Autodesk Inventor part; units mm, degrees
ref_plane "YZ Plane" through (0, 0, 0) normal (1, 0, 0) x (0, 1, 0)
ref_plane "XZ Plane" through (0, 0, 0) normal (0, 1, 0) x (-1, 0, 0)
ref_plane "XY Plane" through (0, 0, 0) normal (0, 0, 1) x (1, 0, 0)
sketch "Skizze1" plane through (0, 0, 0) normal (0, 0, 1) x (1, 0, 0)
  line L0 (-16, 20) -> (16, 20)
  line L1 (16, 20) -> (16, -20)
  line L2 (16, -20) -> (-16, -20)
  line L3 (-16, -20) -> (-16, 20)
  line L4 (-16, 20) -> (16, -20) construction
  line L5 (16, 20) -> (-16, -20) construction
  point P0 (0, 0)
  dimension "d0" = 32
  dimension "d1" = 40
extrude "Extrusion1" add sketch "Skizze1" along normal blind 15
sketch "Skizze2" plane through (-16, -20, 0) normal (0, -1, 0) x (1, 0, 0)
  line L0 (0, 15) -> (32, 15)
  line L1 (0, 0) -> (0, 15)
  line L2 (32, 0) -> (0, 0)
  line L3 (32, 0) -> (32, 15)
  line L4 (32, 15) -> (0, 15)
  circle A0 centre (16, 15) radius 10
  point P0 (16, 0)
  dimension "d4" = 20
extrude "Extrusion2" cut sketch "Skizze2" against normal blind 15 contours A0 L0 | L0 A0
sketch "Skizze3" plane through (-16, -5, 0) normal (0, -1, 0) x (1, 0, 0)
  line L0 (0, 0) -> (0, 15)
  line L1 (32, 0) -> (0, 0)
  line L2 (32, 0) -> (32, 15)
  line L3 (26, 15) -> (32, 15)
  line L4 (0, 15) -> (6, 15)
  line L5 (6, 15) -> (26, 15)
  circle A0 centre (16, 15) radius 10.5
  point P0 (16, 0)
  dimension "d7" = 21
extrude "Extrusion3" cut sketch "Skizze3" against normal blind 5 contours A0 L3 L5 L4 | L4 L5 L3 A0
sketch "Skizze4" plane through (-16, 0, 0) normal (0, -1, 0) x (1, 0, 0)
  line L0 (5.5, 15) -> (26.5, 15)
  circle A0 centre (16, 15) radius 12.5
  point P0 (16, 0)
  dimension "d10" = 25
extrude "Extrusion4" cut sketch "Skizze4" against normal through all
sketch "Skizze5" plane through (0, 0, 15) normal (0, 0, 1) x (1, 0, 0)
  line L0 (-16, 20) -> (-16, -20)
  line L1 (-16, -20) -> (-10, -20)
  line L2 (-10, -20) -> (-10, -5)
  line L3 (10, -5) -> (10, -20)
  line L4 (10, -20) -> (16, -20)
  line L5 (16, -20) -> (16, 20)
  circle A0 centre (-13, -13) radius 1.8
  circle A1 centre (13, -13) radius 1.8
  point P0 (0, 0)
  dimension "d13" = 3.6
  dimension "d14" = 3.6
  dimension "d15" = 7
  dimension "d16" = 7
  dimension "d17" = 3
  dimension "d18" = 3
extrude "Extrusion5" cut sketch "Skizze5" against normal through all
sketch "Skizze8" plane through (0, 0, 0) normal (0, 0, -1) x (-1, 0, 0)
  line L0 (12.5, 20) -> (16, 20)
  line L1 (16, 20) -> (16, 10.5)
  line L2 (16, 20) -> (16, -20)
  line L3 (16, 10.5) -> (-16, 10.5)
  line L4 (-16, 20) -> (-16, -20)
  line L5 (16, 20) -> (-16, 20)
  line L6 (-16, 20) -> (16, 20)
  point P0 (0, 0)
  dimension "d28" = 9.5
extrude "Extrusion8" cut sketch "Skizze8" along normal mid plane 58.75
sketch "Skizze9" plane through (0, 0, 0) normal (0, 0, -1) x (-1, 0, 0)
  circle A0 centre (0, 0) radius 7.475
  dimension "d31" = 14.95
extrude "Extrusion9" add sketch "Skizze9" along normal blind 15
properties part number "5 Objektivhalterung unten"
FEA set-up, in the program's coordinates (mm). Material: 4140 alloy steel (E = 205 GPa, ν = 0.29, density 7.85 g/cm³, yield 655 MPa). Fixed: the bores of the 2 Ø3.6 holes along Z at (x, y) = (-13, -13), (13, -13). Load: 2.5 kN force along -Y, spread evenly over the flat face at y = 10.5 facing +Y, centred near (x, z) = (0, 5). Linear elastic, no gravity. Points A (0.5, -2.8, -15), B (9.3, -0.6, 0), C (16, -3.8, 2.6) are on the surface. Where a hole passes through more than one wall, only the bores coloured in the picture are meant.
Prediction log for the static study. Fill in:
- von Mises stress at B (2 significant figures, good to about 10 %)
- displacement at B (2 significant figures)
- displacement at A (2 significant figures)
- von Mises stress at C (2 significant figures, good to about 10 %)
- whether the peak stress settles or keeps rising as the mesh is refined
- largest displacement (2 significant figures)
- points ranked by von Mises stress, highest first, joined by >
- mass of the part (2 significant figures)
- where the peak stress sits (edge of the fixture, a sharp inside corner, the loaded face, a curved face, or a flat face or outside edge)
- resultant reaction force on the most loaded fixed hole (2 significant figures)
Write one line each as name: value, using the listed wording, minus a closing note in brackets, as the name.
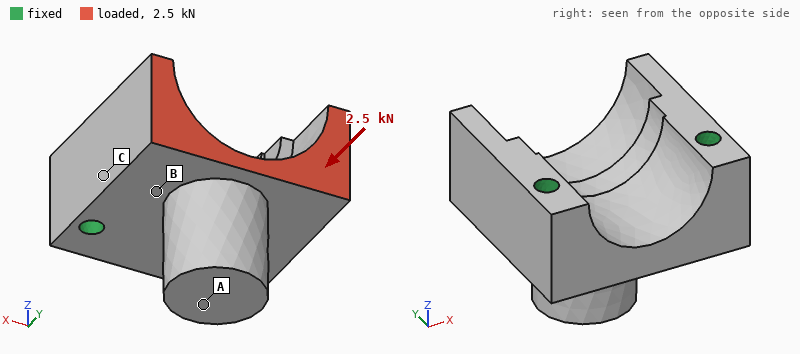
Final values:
von Mises stress at B: 8.9 MPa
displacement at B: 0.96 µm
displacement at A: 1.6 µm
von Mises stress at C: 14 MPa
whether the peak stress settles or keeps rising as the mesh is refined: keeps rising
largest displacement: 1.7 µm
points ranked by von Mises stress, highest first, joined by >: C > B > A
mass of the part: 88 g
where the peak stress sits: edge of the fixture
resultant reaction force on the most loaded fixed hole: 1.3 kN
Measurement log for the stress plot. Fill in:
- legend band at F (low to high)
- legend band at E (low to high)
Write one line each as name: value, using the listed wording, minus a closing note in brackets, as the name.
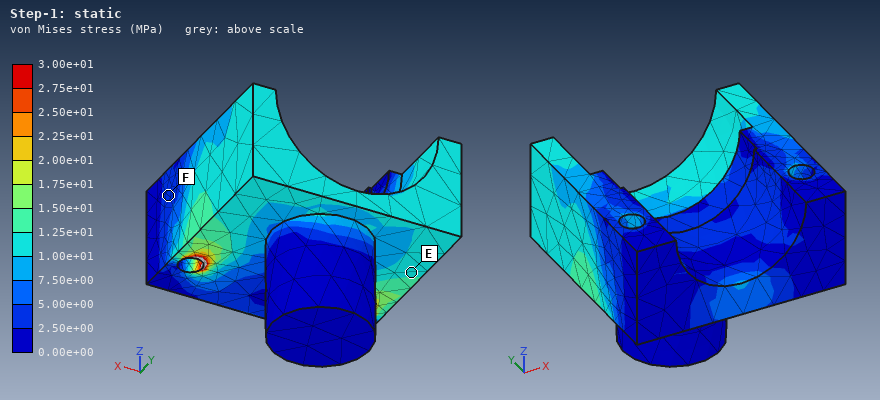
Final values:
legend band at F: 2.50e+00 to 5.00e+00 MPa
legend band at E: 1.00e+01 to 1.25e+01 MPa
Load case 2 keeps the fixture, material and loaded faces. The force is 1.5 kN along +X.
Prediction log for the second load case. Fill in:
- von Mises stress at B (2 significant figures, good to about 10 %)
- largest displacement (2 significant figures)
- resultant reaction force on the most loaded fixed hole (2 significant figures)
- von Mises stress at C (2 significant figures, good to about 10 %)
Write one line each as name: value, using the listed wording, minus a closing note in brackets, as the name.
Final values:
von Mises stress at B: 10 MPa
largest displacement: 9.9 µm
resultant reaction force on the most loaded fixed hole: 1.4 kN
von Mises stress at C: 28 MPa
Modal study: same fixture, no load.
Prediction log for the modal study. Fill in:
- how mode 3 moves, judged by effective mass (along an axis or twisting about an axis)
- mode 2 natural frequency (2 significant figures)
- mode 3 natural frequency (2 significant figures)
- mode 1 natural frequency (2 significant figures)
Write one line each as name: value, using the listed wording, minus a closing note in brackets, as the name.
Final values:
how mode 3 moves, judged by effective mass: along X
mode 2 natural frequency: 16 kHz
mode 3 natural frequency: 19 kHz
mode 1 natural frequency: 11 kHz
